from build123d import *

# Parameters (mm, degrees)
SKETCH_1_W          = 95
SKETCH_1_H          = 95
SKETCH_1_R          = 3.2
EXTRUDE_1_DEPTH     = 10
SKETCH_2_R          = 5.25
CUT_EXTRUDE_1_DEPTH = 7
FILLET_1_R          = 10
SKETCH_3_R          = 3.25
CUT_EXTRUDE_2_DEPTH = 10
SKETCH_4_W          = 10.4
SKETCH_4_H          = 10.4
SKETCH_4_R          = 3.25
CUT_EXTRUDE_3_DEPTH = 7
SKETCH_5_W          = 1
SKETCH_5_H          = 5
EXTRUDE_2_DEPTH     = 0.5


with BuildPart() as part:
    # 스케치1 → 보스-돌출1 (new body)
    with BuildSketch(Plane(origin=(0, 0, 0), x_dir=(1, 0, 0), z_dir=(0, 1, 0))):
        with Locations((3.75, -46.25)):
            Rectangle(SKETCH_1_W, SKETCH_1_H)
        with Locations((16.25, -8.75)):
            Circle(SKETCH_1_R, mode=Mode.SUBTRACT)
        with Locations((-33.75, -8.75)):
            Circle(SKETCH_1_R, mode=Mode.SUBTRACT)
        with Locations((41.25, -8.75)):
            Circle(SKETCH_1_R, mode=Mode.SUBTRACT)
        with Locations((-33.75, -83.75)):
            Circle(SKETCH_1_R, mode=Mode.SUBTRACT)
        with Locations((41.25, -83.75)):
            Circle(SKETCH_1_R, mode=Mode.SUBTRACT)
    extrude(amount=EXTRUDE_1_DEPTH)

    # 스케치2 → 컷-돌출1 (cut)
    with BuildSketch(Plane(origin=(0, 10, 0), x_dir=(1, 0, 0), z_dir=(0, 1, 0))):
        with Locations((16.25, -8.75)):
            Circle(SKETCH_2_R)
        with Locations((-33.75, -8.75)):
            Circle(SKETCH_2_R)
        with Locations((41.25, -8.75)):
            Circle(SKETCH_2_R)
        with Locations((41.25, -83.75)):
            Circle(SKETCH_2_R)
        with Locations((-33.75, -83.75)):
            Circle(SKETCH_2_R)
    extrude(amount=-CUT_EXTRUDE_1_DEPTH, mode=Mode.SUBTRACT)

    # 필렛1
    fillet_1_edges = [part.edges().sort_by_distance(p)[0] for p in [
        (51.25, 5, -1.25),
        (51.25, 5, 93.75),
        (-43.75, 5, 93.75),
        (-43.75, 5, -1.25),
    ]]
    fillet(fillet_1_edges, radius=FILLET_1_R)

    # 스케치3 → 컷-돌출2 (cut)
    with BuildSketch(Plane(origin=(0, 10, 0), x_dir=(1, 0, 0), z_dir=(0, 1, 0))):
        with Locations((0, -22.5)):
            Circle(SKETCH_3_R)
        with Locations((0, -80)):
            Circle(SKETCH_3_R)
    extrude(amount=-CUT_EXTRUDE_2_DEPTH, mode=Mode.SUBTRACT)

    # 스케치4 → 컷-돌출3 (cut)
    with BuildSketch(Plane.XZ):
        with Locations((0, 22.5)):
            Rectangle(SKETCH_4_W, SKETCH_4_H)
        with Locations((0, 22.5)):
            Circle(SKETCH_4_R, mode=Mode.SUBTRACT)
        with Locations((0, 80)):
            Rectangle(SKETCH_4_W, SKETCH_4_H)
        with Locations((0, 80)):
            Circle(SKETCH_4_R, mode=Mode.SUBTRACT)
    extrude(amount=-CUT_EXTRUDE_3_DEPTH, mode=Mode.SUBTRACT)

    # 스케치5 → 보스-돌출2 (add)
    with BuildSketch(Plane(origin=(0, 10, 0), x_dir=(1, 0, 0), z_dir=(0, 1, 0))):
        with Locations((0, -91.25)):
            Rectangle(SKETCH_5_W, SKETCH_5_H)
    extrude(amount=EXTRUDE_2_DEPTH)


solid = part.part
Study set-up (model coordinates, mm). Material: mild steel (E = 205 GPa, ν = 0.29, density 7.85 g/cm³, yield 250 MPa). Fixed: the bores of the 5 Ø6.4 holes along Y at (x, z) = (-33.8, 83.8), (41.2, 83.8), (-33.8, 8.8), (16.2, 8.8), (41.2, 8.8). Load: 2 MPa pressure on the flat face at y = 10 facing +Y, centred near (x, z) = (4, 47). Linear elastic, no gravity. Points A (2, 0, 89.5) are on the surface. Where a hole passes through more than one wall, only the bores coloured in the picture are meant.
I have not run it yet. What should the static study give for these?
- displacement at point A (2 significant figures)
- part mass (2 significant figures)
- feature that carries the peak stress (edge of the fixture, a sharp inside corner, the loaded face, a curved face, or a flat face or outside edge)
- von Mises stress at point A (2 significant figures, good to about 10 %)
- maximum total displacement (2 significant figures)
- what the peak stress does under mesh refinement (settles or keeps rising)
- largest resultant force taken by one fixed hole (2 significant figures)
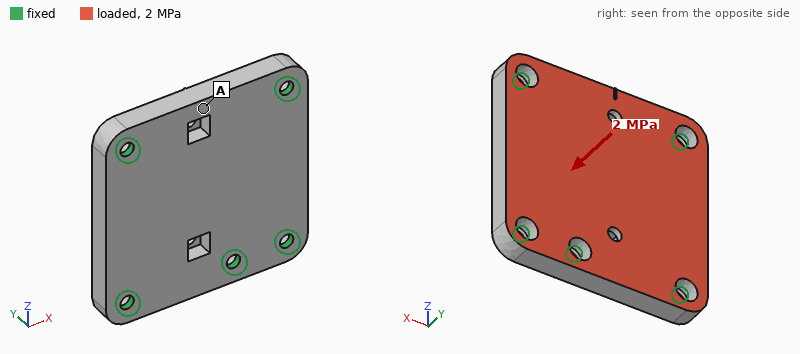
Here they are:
23 µm
660 g
edge of the fixture
49 MPa
35 µm
keeps rising
6.2 kN
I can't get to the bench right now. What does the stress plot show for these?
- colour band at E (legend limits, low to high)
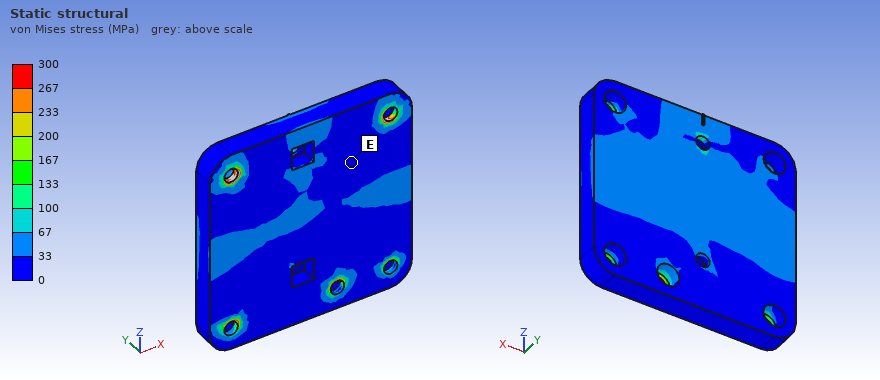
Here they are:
0 to 33 MPa
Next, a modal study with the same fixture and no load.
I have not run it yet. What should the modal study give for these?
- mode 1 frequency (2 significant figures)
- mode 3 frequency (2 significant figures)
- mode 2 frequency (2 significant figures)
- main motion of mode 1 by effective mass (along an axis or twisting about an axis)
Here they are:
5100 Hz
7400 Hz
7200 Hz
along Y
